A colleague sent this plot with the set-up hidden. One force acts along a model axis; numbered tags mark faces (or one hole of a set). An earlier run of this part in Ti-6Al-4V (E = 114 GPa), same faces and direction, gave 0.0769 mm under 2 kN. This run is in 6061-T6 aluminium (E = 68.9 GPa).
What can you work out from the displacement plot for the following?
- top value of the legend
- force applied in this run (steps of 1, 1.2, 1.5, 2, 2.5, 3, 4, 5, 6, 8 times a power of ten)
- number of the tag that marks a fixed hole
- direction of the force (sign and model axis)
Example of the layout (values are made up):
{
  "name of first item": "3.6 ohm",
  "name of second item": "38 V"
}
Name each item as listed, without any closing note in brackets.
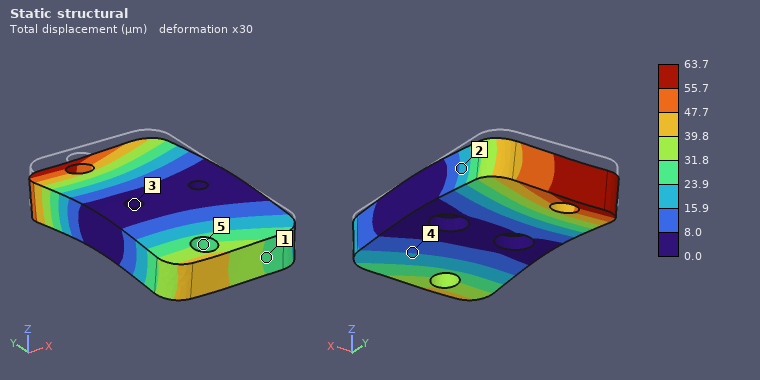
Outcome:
{
  "top value of the legend": "63.7 µm",
  "force applied in this run": "1 kN",
  "number of the tag that marks a fixed hole": "3",
  "direction of the force": "-Z"
}
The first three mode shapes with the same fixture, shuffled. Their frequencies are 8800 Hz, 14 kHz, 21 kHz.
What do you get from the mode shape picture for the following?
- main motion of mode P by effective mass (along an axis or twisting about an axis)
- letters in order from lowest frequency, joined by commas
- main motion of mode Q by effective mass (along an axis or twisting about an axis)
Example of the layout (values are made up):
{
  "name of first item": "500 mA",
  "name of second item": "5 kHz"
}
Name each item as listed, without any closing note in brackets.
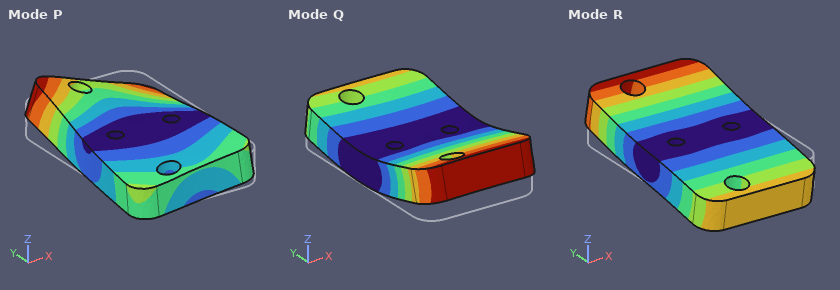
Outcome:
{
  "main motion of mode P by effective mass": "twisting about Z",
  "letters in order from lowest frequency, joined by commas": "R, Q, P",
  "main motion of mode Q by effective mass": "along Z"
}
